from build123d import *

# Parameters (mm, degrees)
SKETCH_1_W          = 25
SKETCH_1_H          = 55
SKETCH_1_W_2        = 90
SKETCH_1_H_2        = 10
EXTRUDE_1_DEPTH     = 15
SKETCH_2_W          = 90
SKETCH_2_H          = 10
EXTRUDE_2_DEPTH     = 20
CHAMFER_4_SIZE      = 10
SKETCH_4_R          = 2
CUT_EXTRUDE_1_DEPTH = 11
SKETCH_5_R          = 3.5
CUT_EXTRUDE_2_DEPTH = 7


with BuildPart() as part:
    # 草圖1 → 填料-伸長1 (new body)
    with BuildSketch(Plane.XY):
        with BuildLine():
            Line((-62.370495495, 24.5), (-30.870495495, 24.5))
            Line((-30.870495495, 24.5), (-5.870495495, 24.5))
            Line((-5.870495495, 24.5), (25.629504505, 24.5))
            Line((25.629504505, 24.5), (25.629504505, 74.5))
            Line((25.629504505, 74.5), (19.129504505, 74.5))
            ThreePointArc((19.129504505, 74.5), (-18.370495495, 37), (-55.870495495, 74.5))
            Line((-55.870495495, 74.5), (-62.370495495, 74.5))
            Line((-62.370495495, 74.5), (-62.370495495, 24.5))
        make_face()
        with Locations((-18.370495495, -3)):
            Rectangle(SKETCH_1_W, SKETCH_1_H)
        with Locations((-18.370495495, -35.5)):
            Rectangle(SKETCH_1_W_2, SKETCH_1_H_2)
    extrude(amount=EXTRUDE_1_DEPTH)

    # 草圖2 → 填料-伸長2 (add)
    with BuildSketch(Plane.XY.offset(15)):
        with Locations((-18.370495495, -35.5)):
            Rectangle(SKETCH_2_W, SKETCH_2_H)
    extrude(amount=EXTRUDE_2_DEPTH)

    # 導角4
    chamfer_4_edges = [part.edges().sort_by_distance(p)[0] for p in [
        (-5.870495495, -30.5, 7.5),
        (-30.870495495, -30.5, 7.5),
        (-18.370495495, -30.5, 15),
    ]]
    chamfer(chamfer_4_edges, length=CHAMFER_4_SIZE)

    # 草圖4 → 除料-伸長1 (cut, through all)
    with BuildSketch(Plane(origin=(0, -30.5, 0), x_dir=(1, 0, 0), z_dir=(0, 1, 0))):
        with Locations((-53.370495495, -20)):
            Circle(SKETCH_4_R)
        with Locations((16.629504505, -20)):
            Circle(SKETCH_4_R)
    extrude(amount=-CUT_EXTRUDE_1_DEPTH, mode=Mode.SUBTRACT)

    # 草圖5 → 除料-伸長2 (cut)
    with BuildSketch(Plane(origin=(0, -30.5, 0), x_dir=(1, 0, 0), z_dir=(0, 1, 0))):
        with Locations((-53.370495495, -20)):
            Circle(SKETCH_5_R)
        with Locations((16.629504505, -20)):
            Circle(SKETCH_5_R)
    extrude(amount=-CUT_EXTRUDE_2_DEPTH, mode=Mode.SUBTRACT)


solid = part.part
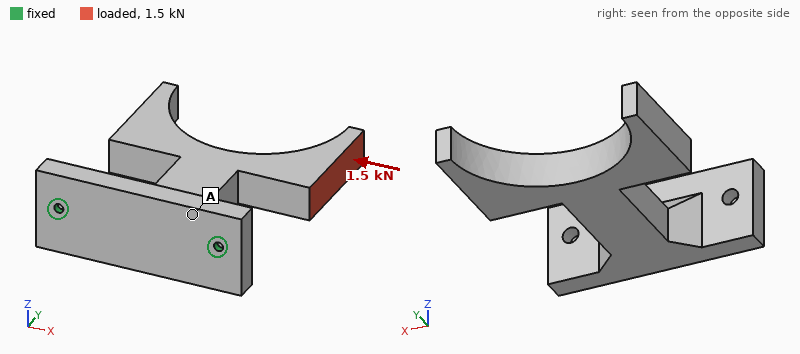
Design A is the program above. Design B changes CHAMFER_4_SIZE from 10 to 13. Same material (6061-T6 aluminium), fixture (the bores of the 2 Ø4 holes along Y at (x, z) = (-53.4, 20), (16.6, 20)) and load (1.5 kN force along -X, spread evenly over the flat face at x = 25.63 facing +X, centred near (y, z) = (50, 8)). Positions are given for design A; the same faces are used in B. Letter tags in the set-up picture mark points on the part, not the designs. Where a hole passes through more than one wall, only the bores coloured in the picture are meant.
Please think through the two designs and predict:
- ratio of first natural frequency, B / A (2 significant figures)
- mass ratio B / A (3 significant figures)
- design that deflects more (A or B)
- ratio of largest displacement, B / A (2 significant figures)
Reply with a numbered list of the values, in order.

1. 1.0
2. 1.03
3. A
4. 0.89
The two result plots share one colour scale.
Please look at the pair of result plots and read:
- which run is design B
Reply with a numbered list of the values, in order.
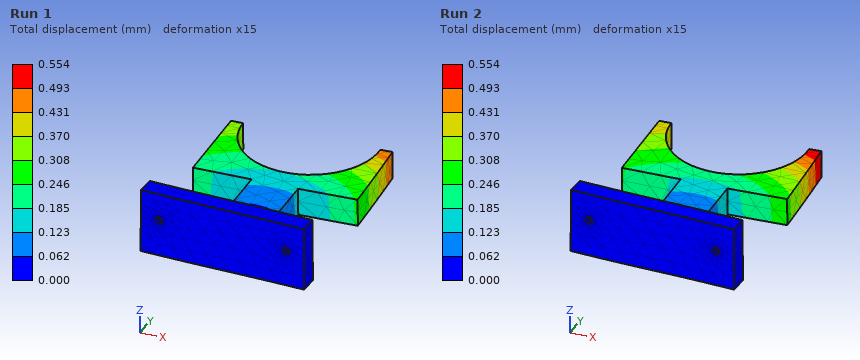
1. Run 1
